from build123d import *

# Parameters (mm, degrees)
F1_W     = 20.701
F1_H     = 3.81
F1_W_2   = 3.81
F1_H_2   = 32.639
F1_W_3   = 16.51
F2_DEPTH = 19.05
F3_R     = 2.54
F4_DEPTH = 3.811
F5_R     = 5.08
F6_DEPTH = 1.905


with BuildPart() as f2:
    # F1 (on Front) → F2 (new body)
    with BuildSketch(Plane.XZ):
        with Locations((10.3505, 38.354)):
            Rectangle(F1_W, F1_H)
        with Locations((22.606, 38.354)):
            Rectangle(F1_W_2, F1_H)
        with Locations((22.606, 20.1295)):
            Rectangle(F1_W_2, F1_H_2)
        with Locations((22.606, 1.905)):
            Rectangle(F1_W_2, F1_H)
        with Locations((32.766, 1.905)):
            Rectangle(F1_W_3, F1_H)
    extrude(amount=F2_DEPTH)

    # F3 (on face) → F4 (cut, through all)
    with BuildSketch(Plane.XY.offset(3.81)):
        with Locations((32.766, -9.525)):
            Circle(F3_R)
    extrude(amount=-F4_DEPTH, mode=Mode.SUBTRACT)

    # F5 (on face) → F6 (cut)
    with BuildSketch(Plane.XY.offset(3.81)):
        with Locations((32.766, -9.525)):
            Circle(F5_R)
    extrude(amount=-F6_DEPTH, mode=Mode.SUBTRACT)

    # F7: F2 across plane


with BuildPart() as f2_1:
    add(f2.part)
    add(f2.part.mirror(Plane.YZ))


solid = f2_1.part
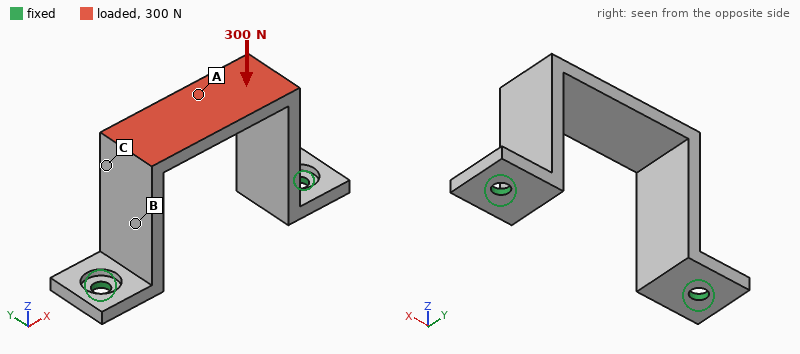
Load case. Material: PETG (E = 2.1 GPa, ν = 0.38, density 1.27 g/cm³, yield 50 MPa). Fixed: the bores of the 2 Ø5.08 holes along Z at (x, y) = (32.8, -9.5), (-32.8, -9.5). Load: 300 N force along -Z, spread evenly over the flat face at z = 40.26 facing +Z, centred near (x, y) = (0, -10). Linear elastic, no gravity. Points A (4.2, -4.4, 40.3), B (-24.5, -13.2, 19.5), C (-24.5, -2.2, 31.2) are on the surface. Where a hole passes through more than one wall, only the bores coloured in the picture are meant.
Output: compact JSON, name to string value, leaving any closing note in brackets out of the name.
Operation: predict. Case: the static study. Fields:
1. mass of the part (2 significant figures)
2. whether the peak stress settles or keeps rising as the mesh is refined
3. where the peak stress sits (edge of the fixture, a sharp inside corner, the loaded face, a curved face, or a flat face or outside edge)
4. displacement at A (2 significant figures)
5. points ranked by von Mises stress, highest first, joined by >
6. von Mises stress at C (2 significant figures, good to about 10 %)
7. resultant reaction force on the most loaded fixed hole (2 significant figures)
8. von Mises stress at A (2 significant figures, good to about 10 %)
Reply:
{"mass of the part": "14 g", "whether the peak stress settles or keeps rising as the mesh is refined": "keeps rising", "where the peak stress sits": "edge of the fixture", "displacement at A": "0.84 mm", "points ranked by von Mises stress, highest first, joined by >": "A > C > B", "von Mises stress at C": "9.7 MPa", "resultant reaction force on the most loaded fixed hole": "160 N", "von Mises stress at A": "14 MPa"}
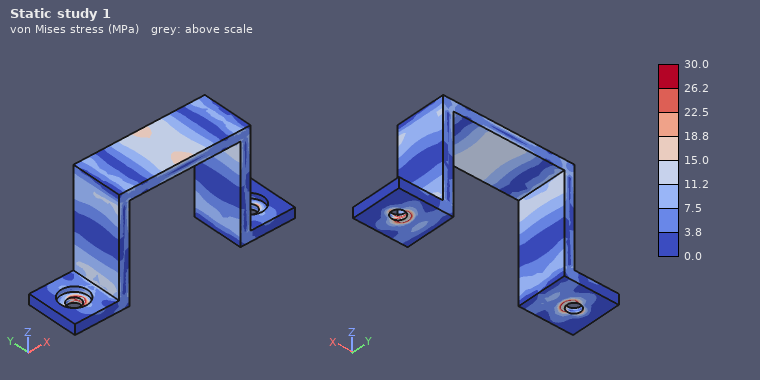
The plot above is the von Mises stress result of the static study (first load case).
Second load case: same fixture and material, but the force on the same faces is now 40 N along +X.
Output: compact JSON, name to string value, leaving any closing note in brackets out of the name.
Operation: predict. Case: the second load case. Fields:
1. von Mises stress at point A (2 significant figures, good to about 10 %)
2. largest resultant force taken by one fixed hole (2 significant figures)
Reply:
{"von Mises stress at point A": "1.7 MPa", "largest resultant force taken by one fixed hole": "28 N"}
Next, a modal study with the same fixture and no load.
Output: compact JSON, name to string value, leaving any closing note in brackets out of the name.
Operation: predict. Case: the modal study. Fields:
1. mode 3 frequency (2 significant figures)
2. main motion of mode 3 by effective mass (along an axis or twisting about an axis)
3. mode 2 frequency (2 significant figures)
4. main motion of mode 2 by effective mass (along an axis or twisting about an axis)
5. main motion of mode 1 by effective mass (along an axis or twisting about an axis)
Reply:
{"mode 3 frequency": "630 Hz", "main motion of mode 3 by effective mass": "twisting about Z", "mode 2 frequency": "400 Hz", "main motion of mode 2 by effective mass": "along X", "main motion of mode 1 by effective mass": "along Y"}
